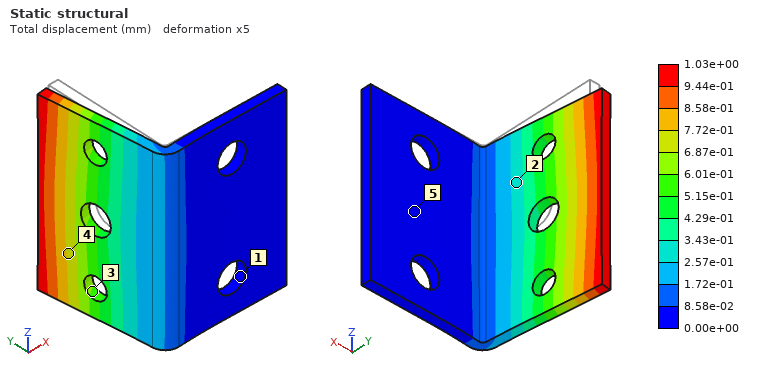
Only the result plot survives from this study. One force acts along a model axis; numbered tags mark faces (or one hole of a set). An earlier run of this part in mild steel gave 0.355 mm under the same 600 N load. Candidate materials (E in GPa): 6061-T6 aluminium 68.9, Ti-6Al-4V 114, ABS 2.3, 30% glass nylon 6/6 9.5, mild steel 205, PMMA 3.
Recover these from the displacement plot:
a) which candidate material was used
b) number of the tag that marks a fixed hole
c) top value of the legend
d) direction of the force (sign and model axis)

6061-T6 aluminium
1
1.03e+00 mm
-X
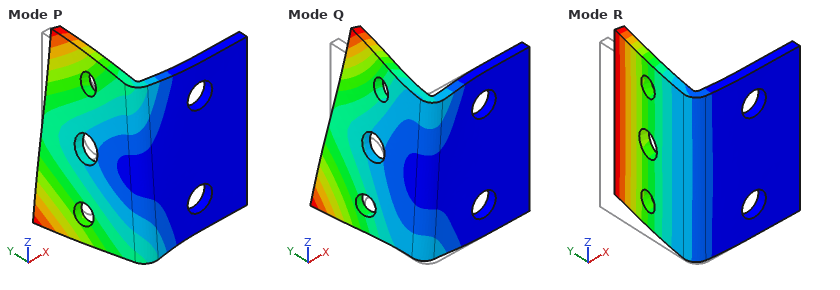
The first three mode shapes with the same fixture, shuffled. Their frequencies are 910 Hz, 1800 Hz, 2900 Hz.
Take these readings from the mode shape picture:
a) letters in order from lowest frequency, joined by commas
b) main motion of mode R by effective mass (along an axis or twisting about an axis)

R, P, Q
along X
